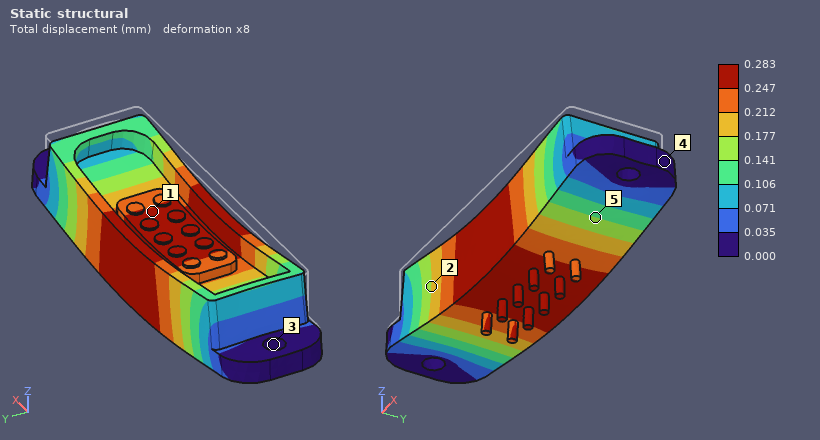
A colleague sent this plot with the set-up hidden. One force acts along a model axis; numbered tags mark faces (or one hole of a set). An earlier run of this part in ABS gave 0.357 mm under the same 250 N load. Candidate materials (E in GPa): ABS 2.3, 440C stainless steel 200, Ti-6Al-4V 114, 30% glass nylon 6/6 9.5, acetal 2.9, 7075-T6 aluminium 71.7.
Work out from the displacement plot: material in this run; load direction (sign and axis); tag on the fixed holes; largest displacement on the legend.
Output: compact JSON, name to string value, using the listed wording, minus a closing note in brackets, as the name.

{"material in this run": "acetal", "load direction": "-Z", "tag on the fixed holes": "3", "largest displacement on the legend": "0.283 mm"}
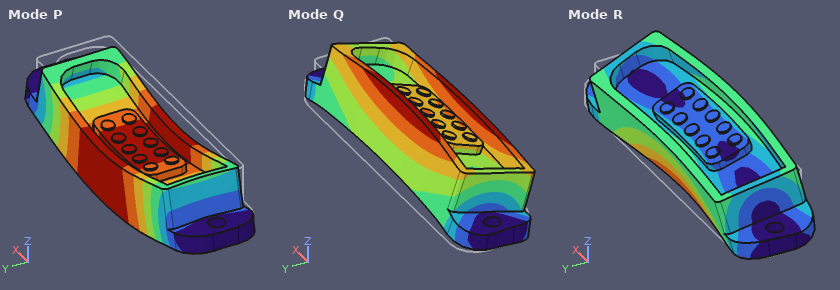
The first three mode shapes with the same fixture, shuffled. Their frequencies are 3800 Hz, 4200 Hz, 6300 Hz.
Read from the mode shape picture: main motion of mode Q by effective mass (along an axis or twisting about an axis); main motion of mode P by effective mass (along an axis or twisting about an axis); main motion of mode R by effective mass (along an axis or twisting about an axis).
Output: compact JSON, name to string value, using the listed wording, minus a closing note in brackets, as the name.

{"main motion of mode Q by effective mass": "along Y", "main motion of mode P by effective mass": "along Z", "main motion of mode R by effective mass": "along Y"}
